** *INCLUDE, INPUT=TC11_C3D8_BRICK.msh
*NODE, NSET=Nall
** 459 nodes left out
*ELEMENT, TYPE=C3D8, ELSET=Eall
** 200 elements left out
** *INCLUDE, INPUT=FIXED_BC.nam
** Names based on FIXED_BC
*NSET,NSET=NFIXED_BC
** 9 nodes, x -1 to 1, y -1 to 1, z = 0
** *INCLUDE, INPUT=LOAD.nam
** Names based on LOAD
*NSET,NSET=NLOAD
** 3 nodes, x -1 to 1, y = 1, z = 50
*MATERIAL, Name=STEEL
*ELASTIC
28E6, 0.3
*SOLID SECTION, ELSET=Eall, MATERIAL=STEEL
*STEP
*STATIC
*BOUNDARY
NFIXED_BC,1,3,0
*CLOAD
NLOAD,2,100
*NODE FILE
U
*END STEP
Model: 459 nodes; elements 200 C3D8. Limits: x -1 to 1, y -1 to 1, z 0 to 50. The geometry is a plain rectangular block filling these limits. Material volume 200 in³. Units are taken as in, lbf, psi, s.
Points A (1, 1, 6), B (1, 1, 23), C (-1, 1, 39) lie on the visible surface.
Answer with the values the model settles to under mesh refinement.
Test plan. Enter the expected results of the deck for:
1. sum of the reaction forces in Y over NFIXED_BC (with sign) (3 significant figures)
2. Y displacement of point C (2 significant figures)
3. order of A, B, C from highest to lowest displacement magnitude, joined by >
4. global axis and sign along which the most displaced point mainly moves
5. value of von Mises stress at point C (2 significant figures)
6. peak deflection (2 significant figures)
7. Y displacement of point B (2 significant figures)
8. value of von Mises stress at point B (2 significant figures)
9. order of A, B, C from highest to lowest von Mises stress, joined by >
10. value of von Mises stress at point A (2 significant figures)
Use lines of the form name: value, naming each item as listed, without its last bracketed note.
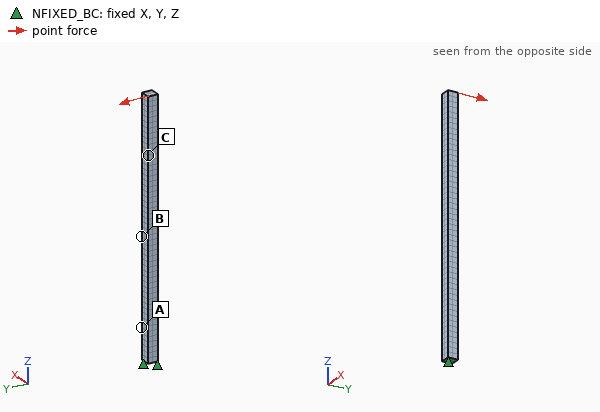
sum of the reaction forces in Y over NFIXED_BC (with sign): -300 lbf
Y displacement of point C: 0.23 in
order of A, B, C from highest to lowest displacement magnitude, joined by >: C > B > A
global axis and sign along which the most displaced point mainly moves: +Y
value of von Mises stress at point C: 2500 psi
peak deflection: 0.33 in
Y displacement of point B: 0.090 in
value of von Mises stress at point B: 6100 psi
order of A, B, C from highest to lowest von Mises stress, joined by >: A > B > C
value of von Mises stress at point A: 9900 psi
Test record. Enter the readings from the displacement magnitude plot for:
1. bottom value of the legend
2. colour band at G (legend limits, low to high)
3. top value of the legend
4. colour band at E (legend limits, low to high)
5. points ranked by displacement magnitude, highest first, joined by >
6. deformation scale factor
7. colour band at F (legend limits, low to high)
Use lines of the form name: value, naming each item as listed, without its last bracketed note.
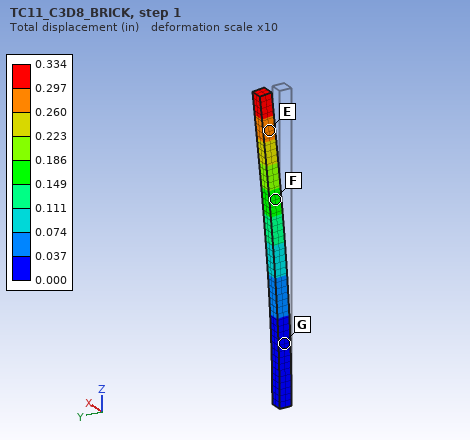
bottom value of the legend: 0.000 in
colour band at G: 0.000 to 0.037 in
top value of the legend: 0.334 in
colour band at E: 0.260 to 0.297 in
points ranked by displacement magnitude, highest first, joined by >: E > F > G
deformation scale factor: 10
colour band at F: 0.149 to 0.186 in
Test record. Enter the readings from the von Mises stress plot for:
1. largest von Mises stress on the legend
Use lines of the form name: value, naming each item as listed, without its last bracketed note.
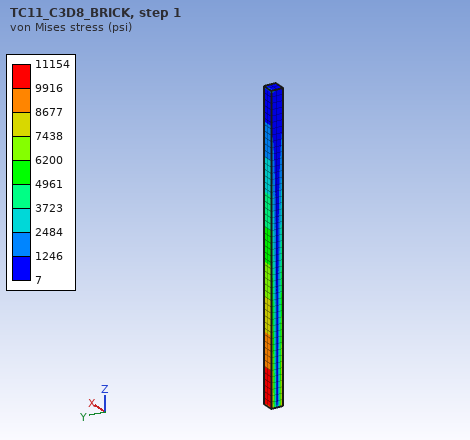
largest von Mises stress on the legend: 11154 psi
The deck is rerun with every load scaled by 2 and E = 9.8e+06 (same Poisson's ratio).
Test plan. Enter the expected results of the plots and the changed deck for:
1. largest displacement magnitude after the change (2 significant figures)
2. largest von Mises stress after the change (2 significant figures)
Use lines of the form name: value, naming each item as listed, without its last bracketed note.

largest displacement magnitude after the change: 1.9 in
largest von Mises stress after the change: 22000 psi
